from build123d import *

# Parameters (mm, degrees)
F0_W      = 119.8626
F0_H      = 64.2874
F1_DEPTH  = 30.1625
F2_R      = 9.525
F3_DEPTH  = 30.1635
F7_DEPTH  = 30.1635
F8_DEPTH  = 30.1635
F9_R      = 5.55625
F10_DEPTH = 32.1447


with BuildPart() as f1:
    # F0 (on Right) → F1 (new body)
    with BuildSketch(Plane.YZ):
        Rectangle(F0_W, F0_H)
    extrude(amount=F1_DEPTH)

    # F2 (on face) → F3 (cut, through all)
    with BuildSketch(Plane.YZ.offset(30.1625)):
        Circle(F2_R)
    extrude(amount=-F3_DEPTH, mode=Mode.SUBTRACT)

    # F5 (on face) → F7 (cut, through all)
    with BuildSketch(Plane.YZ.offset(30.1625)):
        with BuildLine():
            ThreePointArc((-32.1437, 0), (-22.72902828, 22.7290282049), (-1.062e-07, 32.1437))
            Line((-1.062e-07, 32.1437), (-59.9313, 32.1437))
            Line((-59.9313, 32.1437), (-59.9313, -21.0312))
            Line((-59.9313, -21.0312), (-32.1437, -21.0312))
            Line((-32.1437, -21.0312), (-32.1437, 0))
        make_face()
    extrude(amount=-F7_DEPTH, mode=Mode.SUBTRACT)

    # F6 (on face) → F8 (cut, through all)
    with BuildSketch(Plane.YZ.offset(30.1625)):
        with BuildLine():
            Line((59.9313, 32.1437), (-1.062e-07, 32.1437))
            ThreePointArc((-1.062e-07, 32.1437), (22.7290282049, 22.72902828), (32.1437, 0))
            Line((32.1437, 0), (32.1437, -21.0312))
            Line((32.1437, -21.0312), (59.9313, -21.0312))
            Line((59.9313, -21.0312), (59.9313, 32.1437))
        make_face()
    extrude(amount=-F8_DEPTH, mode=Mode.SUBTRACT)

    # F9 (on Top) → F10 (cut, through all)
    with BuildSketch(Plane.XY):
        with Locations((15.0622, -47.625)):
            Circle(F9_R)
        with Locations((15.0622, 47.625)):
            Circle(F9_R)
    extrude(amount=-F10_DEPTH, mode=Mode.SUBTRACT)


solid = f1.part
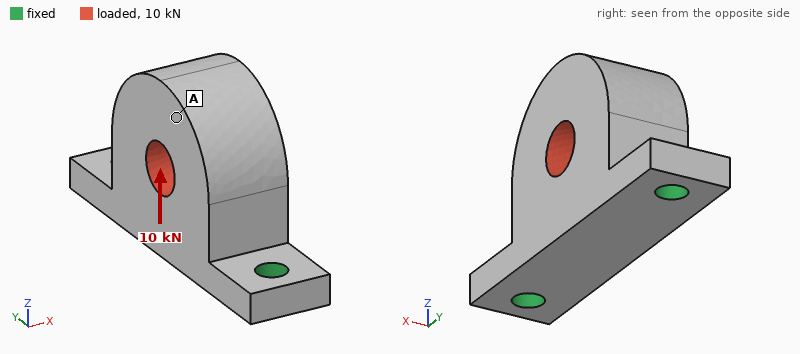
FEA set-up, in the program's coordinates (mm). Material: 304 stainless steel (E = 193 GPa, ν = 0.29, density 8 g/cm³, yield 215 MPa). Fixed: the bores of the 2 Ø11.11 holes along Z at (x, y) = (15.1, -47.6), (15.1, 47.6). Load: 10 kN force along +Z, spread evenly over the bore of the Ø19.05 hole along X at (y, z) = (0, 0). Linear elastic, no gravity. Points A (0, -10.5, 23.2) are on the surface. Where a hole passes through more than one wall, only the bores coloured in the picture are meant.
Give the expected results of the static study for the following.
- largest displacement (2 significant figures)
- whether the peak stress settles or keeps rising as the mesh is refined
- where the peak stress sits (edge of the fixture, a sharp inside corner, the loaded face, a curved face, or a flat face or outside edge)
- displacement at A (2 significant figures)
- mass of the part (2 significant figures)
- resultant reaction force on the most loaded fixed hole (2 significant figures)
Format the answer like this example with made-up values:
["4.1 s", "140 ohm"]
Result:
["11 µm", "keeps rising", "edge of the fixture", "9.8 µm", "950 g", "5.6 kN"]
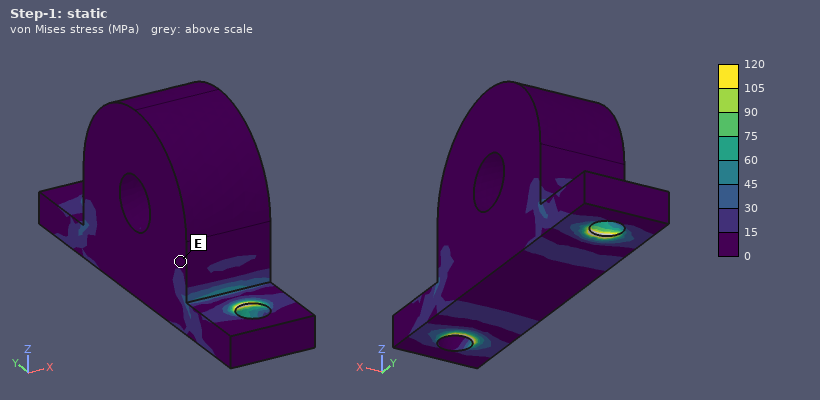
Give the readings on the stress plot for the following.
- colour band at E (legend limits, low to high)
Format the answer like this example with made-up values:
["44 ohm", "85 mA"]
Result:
["0 to 15 MPa"]
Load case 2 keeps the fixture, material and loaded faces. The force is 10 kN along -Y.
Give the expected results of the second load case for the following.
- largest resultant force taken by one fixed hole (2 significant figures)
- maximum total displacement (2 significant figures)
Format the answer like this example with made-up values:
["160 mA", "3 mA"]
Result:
["6.1 kN", "12 µm"]
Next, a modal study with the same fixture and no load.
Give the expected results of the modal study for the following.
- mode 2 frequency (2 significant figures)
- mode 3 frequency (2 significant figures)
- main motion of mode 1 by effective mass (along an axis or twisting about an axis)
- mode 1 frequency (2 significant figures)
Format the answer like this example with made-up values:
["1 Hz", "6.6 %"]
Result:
["5700 Hz", "5900 Hz", "along X", "1900 Hz"]
